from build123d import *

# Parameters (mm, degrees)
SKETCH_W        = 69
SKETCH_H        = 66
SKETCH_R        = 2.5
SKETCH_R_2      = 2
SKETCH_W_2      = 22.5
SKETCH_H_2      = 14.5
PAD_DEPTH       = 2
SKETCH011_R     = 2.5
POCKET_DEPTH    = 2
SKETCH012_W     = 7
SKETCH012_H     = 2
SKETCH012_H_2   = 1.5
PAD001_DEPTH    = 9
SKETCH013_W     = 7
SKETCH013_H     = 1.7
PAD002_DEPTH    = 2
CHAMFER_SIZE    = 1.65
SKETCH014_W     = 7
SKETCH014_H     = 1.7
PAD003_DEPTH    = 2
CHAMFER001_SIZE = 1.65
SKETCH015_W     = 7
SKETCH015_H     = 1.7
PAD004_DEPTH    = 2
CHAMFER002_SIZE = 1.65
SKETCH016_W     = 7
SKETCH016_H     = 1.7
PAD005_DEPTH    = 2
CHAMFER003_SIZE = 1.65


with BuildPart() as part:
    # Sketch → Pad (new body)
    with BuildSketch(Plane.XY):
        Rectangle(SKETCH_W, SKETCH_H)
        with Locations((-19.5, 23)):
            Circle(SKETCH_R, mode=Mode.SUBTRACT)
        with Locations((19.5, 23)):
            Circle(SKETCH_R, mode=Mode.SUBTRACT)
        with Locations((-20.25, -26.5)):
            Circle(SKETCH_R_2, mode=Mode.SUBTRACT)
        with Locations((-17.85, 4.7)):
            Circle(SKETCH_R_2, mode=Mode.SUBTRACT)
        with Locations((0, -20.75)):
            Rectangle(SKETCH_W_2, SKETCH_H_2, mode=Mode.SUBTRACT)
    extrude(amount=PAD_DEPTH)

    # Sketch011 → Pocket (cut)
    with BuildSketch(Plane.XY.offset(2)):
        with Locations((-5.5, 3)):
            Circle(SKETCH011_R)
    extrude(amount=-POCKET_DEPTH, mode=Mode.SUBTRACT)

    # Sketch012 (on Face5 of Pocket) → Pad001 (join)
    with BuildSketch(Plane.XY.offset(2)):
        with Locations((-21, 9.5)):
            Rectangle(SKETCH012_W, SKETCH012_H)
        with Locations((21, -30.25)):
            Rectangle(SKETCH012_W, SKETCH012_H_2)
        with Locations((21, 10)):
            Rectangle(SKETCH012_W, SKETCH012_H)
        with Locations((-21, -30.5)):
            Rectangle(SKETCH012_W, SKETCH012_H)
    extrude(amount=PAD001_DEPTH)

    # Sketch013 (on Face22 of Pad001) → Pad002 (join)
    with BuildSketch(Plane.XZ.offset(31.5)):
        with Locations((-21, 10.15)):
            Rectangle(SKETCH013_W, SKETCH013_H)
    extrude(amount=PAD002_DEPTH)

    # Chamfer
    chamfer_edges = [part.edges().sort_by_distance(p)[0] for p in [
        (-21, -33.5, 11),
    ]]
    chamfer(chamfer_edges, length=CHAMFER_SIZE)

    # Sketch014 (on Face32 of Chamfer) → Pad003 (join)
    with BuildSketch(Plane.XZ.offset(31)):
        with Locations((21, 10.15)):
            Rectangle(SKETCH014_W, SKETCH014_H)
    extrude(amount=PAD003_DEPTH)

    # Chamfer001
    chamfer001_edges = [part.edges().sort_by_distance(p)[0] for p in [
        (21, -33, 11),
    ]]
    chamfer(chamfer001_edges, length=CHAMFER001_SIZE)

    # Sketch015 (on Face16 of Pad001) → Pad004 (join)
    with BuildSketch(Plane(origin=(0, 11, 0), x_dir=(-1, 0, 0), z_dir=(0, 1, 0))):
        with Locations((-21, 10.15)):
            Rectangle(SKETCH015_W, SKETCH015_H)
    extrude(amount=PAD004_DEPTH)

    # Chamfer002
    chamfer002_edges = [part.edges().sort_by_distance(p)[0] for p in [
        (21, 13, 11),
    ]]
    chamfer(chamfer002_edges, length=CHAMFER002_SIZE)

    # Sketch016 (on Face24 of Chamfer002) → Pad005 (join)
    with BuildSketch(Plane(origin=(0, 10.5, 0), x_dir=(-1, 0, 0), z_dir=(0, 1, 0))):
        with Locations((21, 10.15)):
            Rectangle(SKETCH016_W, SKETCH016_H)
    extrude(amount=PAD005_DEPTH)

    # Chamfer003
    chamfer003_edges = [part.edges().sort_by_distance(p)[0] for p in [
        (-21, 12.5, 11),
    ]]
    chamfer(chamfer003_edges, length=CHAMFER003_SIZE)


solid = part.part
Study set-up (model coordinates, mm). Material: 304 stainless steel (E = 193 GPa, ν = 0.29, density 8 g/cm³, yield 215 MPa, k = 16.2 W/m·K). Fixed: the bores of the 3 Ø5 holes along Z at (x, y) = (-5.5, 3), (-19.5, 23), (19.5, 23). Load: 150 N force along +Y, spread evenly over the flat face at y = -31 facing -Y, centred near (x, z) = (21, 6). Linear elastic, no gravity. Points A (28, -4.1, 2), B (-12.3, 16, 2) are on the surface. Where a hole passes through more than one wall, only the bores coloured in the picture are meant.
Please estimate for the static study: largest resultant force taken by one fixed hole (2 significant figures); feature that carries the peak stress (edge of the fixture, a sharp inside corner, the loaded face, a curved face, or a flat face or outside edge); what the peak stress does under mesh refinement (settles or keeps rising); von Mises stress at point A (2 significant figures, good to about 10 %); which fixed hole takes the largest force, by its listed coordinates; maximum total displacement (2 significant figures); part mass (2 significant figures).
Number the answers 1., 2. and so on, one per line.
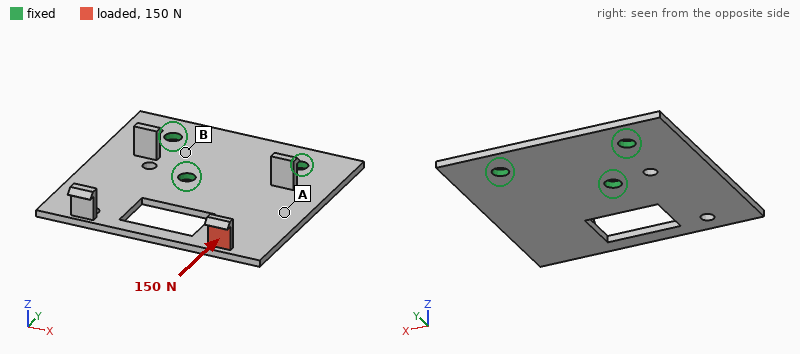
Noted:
1. 120 N
2. a sharp inside corner
3. keeps rising
4. 25 MPa
5. (19.5, 23)
6. 0.15 mm
7. 71 g
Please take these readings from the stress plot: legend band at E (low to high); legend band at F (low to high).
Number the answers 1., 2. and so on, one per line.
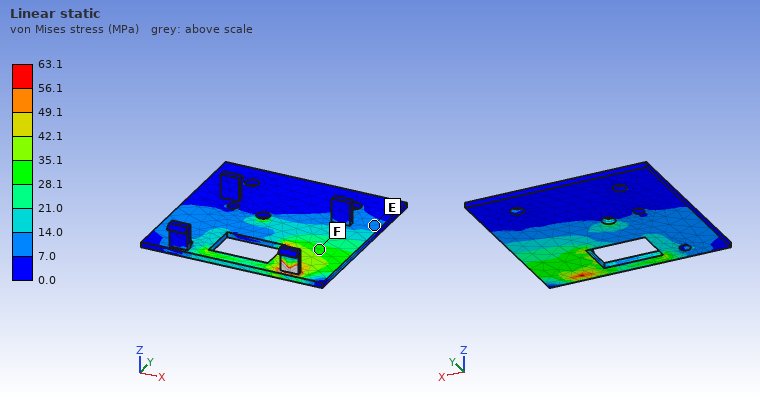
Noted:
1. 7.0 to 14.0 MPa
2. 28.1 to 35.1 MPa
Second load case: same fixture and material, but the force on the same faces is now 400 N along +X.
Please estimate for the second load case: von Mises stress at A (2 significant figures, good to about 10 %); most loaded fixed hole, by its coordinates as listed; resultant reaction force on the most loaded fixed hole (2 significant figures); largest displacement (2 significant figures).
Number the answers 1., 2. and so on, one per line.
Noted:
1. 55 MPa
2. (-5.5, 3)
3. 520 N
4. 0.31 mm
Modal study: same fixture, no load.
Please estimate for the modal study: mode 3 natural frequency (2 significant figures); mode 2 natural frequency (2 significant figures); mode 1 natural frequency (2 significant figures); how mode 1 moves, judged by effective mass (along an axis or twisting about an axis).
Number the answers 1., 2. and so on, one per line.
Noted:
1. 2600 Hz
2. 1100 Hz
3. 870 Hz
4. along Z
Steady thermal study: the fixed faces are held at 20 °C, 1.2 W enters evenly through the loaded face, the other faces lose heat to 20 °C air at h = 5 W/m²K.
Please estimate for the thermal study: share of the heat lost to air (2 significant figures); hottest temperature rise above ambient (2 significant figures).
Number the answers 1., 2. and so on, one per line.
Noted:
1. 35 %
2. 73 K
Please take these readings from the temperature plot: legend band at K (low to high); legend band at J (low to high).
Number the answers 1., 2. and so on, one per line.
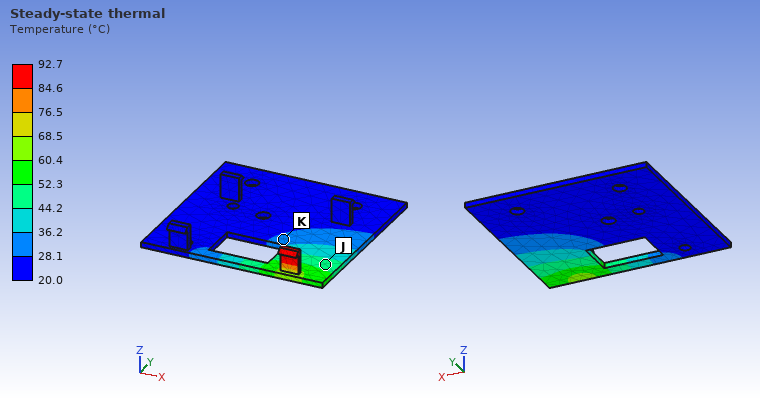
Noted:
1. 28.1 to 36.2 °C
2. 44.2 to 52.3 °C
